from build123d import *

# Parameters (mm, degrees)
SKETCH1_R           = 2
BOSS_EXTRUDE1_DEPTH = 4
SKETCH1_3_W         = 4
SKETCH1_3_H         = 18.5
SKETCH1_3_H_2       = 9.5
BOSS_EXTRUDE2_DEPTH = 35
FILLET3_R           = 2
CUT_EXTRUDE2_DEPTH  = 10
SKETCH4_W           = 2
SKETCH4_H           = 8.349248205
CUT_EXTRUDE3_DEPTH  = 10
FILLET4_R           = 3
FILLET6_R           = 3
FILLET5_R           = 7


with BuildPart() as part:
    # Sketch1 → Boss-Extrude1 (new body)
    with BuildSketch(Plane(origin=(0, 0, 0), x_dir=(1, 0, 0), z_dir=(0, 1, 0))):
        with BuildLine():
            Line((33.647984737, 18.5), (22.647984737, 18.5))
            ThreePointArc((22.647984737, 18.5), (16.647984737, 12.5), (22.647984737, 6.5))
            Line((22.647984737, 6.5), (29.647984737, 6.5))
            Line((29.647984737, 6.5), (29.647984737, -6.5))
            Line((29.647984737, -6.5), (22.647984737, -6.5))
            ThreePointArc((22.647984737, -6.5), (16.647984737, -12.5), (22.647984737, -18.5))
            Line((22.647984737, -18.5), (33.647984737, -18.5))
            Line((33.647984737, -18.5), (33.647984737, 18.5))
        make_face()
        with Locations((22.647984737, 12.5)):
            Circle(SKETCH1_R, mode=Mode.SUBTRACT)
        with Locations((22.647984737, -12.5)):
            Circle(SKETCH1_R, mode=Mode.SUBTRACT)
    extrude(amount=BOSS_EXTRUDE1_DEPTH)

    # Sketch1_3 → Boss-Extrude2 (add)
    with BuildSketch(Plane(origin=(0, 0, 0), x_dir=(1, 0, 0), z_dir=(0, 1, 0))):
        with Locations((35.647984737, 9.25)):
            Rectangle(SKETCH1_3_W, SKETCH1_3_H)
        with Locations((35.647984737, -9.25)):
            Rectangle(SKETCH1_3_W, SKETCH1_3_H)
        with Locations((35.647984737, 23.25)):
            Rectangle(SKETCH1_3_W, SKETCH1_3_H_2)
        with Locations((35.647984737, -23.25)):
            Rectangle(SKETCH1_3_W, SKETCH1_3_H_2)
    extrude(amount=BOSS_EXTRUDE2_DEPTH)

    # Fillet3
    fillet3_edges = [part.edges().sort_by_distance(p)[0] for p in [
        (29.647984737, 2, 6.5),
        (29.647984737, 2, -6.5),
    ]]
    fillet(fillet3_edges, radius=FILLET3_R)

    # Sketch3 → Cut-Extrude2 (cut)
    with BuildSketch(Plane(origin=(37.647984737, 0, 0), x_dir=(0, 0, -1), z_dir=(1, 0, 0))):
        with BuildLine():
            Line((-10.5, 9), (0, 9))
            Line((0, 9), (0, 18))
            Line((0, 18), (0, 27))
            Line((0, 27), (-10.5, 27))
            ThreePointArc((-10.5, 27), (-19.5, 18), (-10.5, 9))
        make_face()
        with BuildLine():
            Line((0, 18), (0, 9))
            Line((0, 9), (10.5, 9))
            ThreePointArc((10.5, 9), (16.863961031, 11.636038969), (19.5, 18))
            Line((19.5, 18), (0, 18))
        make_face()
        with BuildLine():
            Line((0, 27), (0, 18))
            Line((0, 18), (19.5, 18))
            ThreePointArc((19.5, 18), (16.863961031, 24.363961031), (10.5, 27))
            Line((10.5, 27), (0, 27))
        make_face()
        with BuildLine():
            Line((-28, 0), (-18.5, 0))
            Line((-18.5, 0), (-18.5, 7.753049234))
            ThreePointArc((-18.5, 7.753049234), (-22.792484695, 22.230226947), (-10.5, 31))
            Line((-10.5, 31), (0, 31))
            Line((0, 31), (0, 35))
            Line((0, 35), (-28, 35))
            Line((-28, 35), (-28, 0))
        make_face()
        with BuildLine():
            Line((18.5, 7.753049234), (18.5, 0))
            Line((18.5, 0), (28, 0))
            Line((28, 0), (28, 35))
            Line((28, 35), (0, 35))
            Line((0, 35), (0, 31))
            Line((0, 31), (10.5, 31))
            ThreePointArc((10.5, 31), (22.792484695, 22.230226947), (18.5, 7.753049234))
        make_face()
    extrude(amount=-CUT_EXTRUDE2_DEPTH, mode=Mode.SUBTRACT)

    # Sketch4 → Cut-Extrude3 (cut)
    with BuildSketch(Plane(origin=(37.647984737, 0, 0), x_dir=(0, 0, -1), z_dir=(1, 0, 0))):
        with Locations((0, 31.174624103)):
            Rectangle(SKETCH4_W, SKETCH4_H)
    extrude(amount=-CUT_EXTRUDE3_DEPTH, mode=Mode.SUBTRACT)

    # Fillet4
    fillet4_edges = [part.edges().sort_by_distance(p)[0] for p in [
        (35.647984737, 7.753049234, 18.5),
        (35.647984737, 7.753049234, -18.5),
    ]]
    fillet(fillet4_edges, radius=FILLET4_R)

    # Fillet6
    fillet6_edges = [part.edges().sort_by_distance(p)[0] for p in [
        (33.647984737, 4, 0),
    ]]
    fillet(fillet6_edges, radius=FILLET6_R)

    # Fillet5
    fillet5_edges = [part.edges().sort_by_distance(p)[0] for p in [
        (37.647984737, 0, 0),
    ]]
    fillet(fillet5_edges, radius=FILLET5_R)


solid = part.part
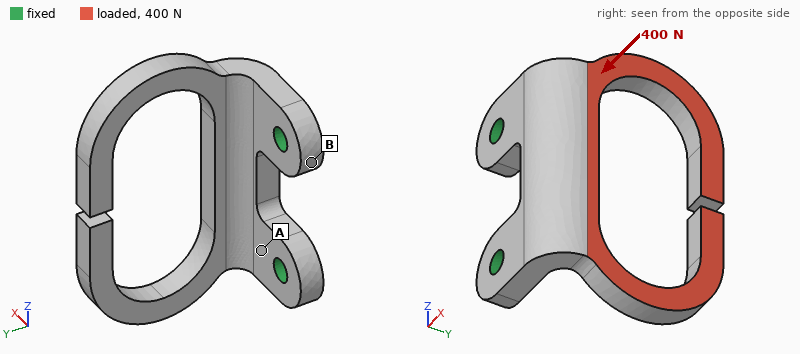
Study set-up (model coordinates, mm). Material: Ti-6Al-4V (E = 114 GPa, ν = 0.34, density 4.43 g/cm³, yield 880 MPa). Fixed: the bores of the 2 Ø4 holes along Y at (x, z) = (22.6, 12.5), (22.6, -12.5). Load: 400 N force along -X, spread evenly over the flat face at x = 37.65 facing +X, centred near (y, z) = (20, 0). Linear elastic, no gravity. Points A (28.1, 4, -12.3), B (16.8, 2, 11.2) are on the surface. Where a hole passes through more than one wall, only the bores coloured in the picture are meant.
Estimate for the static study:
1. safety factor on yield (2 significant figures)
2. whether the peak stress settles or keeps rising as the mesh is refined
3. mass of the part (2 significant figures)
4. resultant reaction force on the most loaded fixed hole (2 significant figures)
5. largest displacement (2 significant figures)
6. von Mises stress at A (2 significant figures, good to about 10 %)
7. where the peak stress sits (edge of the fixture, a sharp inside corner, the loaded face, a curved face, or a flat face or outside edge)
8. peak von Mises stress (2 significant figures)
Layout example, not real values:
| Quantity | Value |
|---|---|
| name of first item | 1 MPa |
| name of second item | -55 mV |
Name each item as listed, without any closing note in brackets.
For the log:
| Quantity | Value |
|---|---|
| safety factor on yield | 3.1 |
| whether the peak stress settles or keeps rising as the mesh is refined | settles |
| mass of the part | 17 g |
| resultant reaction force on the most loaded fixed hole | 200 N |
| largest displacement | 0.63 mm |
| von Mises stress at A | 110 MPa |
| where the peak stress sits | a curved face |
| peak von Mises stress | 280 MPa |
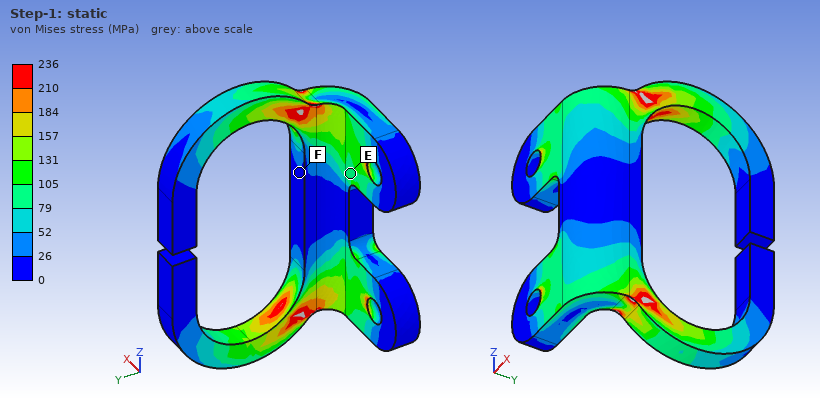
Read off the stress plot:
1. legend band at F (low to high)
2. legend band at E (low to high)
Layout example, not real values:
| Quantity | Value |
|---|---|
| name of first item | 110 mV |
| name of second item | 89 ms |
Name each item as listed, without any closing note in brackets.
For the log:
| Quantity | Value |
|---|---|
| legend band at F | 0 to 26 MPa |
| legend band at E | 79 to 105 MPa |
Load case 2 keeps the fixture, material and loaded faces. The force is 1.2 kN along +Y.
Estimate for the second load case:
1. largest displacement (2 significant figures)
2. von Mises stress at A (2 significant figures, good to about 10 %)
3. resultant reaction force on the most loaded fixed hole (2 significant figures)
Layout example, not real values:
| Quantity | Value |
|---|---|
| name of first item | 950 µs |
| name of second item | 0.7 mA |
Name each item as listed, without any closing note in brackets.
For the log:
| Quantity | Value |
|---|---|
| largest displacement | 0.68 mm |
| von Mises stress at A | 180 MPa |
| resultant reaction force on the most loaded fixed hole | 600 N |
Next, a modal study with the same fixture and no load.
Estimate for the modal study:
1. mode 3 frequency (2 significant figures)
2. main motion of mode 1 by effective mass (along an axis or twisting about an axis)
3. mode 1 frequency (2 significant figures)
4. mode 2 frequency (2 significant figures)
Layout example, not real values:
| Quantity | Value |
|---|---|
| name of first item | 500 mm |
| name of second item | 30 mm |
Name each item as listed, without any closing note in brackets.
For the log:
| Quantity | Value |
|---|---|
| mode 3 frequency | 2500 Hz |
| main motion of mode 1 by effective mass | along X |
| mode 1 frequency | 1900 Hz |
| mode 2 frequency | 2000 Hz |
